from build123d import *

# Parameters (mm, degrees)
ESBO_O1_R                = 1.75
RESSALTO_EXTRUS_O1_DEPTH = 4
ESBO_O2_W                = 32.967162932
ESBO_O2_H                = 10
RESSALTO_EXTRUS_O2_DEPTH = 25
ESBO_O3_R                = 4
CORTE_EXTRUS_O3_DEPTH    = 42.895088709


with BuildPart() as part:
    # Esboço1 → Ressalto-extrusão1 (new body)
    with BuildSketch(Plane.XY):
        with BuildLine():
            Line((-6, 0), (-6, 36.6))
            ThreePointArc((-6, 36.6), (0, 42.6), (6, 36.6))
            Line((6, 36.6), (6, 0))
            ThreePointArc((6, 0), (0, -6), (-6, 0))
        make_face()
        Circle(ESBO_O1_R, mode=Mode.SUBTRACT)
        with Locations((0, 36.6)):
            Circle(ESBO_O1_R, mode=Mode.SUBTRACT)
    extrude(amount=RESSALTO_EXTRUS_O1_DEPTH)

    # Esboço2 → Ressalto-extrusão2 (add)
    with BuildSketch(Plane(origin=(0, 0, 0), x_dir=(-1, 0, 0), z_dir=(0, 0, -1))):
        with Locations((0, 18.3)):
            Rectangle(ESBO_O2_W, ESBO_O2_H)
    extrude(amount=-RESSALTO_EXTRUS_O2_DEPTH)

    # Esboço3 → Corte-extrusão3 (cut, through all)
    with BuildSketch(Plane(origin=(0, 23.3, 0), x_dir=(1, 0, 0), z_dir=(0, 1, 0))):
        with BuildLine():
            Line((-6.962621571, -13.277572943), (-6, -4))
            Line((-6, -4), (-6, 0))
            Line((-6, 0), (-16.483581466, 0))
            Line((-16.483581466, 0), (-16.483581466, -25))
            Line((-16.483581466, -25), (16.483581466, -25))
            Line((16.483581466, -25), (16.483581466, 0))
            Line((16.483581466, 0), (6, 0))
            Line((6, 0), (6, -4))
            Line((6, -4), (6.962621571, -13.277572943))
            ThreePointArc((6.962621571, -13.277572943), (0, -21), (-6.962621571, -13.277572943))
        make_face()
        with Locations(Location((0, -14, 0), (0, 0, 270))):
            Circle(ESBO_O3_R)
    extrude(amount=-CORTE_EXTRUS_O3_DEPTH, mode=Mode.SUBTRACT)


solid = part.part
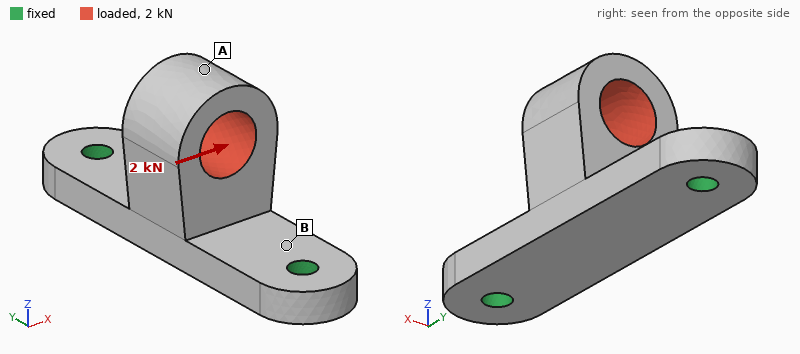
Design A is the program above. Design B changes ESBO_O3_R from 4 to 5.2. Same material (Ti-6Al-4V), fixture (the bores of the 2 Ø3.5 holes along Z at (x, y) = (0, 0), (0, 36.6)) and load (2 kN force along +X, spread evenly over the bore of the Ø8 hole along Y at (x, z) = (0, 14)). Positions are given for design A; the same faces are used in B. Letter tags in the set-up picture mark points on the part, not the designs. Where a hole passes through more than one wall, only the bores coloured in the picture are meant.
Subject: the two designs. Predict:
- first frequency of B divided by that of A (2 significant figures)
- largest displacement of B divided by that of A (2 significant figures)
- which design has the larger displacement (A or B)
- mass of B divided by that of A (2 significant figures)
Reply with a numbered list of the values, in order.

1. 1.1
2. 1.1
3. B
4. 0.91
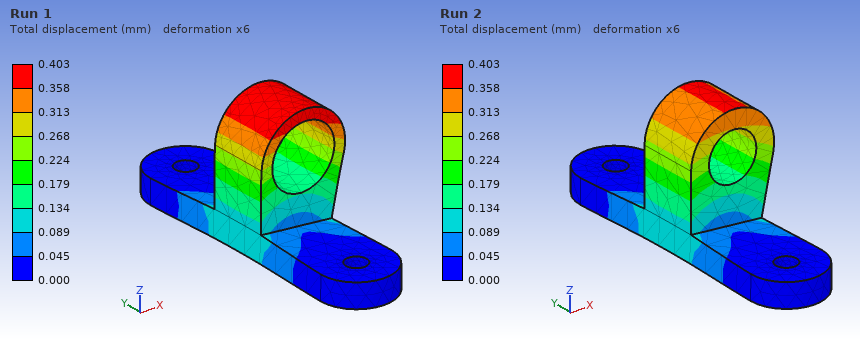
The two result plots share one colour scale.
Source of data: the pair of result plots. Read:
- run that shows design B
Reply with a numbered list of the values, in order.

1. Run 1
